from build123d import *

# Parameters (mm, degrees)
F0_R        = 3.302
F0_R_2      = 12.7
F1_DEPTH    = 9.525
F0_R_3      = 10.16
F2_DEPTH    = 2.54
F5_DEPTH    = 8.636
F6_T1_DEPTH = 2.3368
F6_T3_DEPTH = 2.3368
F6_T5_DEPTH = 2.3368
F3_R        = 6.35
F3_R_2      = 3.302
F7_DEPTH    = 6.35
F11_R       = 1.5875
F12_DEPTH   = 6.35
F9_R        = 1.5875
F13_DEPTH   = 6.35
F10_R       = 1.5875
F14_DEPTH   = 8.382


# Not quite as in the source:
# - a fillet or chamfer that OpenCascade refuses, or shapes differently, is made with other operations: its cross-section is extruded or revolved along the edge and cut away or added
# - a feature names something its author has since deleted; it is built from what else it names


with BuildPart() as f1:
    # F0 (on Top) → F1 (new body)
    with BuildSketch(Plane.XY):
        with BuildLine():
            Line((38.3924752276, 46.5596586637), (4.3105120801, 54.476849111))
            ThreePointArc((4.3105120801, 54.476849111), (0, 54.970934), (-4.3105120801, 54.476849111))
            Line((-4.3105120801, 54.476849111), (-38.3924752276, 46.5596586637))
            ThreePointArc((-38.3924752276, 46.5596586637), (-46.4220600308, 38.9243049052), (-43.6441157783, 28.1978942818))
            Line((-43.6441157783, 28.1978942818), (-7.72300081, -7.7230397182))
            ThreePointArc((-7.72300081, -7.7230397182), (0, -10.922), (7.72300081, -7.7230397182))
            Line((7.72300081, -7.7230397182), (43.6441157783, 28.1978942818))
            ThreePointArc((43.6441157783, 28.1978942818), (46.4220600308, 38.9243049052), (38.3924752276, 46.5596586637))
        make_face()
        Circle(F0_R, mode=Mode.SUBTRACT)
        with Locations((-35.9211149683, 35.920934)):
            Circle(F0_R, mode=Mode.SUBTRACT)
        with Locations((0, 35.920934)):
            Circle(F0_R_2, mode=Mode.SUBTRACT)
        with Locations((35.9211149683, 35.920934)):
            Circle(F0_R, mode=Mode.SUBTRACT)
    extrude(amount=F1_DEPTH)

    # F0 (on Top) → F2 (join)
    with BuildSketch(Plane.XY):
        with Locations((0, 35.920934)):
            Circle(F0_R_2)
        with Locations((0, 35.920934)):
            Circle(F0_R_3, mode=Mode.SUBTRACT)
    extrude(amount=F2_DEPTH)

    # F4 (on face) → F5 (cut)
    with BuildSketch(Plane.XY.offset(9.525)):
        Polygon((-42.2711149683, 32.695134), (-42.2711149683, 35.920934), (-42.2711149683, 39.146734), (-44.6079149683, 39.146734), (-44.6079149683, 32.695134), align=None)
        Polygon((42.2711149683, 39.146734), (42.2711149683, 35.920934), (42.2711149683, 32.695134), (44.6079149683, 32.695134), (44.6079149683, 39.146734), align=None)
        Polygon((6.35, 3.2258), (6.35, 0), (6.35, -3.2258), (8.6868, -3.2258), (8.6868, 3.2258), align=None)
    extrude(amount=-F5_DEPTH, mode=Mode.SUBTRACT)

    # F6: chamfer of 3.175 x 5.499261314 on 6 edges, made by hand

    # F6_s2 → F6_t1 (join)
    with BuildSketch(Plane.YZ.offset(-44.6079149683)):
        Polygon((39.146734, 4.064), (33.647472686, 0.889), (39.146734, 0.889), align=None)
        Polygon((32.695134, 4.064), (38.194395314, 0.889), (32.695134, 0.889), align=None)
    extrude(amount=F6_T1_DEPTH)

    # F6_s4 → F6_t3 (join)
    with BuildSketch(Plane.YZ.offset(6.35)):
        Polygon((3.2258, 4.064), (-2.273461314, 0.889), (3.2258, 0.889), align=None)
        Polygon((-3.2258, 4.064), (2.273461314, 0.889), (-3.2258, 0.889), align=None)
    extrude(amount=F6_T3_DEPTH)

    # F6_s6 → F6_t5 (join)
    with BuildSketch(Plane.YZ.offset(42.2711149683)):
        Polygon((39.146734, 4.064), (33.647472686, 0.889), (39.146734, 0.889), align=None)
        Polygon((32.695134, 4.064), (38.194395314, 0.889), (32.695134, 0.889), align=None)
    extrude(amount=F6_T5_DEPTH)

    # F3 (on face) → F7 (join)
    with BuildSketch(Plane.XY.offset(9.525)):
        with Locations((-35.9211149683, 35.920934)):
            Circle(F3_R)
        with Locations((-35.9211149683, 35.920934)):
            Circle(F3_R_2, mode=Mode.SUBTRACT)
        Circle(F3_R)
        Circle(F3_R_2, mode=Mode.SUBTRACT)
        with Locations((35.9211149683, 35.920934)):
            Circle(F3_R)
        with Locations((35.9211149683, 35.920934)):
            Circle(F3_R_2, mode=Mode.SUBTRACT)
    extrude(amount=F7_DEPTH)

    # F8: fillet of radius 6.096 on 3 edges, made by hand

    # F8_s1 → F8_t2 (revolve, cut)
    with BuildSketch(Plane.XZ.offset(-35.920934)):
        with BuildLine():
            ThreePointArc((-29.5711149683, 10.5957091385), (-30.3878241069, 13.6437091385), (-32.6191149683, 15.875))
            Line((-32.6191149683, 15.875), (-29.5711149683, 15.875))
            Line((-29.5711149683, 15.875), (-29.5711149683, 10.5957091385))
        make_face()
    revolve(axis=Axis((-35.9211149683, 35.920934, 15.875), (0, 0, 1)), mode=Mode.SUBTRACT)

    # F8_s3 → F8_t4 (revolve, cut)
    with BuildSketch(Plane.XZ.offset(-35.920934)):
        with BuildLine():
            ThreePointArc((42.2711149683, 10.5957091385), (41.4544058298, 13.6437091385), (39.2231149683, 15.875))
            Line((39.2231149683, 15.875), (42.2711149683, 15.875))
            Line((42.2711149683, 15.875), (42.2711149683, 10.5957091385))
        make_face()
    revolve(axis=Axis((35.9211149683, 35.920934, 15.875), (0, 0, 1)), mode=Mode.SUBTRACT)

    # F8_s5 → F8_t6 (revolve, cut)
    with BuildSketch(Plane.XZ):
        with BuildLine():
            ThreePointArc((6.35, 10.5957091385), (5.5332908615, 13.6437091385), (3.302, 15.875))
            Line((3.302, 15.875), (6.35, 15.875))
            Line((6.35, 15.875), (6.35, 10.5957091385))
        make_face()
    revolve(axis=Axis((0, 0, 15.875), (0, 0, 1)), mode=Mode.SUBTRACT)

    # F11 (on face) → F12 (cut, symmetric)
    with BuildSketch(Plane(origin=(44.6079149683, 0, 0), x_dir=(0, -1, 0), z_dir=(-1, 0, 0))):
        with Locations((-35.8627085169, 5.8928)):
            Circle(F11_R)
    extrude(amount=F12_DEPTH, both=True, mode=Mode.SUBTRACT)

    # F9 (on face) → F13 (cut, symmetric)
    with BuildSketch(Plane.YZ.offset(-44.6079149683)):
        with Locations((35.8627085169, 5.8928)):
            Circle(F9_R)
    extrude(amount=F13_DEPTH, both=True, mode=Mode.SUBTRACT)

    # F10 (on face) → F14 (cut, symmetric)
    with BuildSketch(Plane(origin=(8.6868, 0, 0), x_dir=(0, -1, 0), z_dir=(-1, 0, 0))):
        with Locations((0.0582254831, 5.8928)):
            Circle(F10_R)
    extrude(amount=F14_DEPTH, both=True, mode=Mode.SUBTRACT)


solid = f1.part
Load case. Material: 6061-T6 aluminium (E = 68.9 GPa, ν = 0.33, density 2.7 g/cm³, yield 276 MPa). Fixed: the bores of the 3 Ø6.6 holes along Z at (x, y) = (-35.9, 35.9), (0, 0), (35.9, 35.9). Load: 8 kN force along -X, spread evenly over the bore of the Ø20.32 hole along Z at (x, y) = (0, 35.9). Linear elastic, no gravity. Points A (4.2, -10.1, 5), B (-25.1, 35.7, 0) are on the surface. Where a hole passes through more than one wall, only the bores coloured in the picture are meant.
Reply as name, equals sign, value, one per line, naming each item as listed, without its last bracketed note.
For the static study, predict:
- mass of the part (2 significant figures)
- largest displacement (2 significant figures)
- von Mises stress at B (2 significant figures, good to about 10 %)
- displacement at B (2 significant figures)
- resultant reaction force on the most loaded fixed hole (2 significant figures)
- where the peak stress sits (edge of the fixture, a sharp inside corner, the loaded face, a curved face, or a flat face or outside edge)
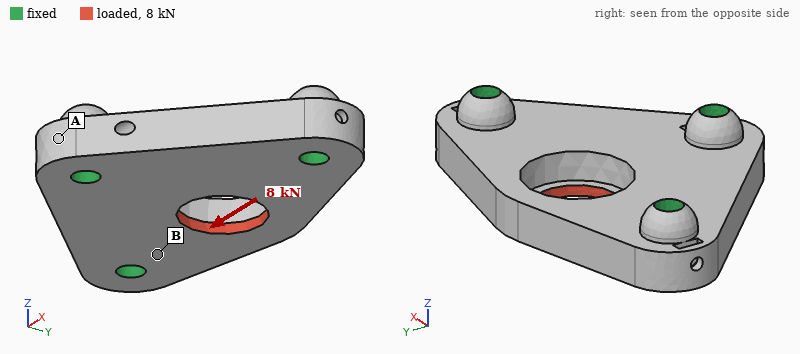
mass of the part = 88 g
largest displacement = 15 µm
von Mises stress at B = 28 MPa
displacement at B = 2.8 µm
resultant reaction force on the most loaded fixed hole = 3.5 kN
where the peak stress sits = a sharp inside corner
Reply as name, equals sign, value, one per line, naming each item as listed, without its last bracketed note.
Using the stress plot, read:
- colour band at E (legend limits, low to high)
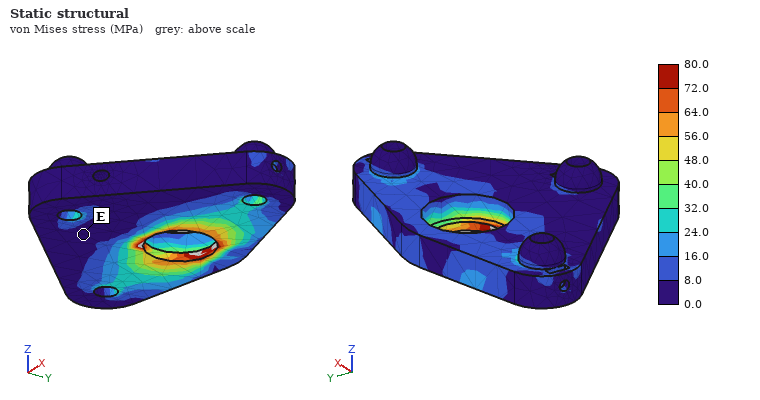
colour band at E = 0.0 to 8.0 MPa
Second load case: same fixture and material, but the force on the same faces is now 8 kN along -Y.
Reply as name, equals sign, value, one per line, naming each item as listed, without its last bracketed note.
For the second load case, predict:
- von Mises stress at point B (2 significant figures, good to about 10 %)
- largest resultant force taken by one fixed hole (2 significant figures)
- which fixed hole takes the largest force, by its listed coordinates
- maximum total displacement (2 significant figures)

von Mises stress at point B = 23 MPa
largest resultant force taken by one fixed hole = 4.2 kN
which fixed hole takes the largest force, by its listed coordinates = (0, 0)
maximum total displacement = 44 µm
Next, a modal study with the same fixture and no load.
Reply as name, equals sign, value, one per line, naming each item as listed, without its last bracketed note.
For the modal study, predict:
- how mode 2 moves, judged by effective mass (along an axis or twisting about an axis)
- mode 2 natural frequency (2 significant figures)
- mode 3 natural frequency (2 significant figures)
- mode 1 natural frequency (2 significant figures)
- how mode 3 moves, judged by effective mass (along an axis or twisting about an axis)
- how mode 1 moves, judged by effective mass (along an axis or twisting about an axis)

how mode 2 moves, judged by effective mass = along Z
mode 2 natural frequency = 17 kHz
mode 3 natural frequency = 18 kHz
mode 1 natural frequency = 9900 Hz
how mode 3 moves, judged by effective mass = twisting about Y
how mode 1 moves, judged by effective mass = along Z
